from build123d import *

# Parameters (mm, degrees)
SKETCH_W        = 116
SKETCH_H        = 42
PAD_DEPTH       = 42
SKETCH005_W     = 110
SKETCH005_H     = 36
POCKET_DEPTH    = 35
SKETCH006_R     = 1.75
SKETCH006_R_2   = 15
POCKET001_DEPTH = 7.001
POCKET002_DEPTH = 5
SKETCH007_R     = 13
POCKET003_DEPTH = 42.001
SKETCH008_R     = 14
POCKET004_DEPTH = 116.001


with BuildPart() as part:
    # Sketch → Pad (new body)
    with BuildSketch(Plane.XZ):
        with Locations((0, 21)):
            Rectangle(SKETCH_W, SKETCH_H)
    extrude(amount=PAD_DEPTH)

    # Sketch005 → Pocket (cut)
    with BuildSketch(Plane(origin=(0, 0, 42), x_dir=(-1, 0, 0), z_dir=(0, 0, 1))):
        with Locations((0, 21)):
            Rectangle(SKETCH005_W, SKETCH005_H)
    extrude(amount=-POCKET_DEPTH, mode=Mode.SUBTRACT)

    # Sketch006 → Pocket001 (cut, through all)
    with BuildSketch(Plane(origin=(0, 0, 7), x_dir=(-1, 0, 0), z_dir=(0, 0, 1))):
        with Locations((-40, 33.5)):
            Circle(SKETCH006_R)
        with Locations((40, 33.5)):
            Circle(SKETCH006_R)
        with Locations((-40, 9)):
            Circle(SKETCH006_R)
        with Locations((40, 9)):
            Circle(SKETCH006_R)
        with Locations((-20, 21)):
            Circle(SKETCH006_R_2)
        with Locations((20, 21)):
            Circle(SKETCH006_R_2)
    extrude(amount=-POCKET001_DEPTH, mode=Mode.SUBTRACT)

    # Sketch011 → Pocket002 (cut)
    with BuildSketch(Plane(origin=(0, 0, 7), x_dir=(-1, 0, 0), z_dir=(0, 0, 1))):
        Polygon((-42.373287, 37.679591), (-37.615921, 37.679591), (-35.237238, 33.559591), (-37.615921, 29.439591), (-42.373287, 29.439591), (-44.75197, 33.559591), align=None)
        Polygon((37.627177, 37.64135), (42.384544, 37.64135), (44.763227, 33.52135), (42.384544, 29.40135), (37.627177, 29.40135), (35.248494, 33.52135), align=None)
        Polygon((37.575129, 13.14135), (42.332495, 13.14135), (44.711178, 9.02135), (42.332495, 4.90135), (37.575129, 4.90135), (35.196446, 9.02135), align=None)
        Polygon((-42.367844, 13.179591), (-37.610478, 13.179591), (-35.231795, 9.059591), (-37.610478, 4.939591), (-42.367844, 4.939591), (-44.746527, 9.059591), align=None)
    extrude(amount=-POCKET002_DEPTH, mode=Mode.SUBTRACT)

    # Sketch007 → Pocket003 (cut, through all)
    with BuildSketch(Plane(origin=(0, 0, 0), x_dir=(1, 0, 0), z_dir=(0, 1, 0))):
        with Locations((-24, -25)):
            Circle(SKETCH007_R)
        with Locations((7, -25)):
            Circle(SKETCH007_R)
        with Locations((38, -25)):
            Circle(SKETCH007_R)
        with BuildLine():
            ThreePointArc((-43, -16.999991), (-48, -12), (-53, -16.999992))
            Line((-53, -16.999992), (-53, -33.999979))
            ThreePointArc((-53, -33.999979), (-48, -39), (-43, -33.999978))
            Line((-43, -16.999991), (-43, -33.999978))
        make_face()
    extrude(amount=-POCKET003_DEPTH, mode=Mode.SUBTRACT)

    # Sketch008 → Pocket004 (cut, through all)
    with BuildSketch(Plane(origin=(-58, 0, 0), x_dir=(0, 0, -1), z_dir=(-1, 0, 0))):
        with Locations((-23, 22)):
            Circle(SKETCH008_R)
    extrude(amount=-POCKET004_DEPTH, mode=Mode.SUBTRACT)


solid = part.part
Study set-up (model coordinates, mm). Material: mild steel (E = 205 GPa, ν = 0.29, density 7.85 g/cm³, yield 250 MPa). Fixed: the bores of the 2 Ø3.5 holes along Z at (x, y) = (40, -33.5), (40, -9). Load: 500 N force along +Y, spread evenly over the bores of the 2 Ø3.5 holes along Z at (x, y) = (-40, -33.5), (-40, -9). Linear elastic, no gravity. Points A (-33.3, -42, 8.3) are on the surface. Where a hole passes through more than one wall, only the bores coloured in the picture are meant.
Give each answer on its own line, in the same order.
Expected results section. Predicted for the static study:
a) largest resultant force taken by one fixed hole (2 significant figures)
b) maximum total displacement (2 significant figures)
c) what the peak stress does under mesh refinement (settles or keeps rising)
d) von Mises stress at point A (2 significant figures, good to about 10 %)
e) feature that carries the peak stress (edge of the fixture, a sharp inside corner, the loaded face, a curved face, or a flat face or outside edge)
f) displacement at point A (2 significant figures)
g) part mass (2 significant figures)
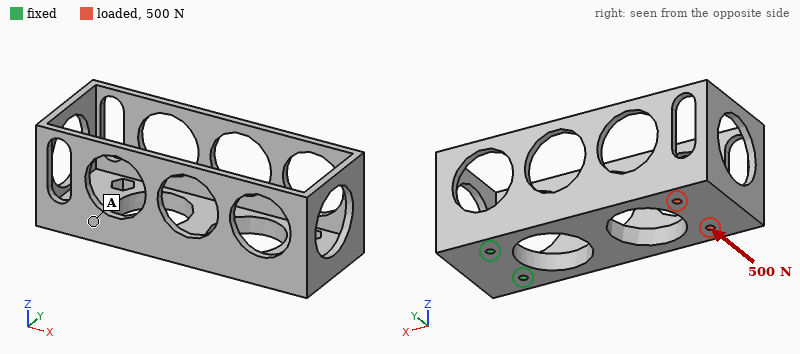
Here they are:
1.5 kN
56 µm
keeps rising
9.4 MPa
edge of the fixture
43 µm
320 g
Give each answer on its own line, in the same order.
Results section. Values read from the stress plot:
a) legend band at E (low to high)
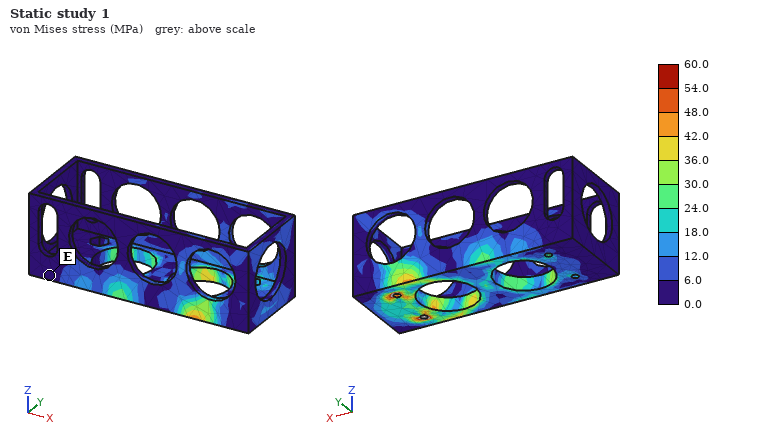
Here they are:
0.0 to 6.0 MPa
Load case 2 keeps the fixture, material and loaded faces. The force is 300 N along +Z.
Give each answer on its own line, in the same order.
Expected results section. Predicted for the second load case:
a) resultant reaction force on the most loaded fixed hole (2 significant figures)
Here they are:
330 N
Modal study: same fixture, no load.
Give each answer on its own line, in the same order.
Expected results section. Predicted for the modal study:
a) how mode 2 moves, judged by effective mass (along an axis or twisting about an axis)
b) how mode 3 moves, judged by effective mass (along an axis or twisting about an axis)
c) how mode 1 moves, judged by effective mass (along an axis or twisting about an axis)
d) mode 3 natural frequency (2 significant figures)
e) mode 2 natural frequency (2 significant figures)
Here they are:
along Y
along Y
along Z
1500 Hz
990 Hz
